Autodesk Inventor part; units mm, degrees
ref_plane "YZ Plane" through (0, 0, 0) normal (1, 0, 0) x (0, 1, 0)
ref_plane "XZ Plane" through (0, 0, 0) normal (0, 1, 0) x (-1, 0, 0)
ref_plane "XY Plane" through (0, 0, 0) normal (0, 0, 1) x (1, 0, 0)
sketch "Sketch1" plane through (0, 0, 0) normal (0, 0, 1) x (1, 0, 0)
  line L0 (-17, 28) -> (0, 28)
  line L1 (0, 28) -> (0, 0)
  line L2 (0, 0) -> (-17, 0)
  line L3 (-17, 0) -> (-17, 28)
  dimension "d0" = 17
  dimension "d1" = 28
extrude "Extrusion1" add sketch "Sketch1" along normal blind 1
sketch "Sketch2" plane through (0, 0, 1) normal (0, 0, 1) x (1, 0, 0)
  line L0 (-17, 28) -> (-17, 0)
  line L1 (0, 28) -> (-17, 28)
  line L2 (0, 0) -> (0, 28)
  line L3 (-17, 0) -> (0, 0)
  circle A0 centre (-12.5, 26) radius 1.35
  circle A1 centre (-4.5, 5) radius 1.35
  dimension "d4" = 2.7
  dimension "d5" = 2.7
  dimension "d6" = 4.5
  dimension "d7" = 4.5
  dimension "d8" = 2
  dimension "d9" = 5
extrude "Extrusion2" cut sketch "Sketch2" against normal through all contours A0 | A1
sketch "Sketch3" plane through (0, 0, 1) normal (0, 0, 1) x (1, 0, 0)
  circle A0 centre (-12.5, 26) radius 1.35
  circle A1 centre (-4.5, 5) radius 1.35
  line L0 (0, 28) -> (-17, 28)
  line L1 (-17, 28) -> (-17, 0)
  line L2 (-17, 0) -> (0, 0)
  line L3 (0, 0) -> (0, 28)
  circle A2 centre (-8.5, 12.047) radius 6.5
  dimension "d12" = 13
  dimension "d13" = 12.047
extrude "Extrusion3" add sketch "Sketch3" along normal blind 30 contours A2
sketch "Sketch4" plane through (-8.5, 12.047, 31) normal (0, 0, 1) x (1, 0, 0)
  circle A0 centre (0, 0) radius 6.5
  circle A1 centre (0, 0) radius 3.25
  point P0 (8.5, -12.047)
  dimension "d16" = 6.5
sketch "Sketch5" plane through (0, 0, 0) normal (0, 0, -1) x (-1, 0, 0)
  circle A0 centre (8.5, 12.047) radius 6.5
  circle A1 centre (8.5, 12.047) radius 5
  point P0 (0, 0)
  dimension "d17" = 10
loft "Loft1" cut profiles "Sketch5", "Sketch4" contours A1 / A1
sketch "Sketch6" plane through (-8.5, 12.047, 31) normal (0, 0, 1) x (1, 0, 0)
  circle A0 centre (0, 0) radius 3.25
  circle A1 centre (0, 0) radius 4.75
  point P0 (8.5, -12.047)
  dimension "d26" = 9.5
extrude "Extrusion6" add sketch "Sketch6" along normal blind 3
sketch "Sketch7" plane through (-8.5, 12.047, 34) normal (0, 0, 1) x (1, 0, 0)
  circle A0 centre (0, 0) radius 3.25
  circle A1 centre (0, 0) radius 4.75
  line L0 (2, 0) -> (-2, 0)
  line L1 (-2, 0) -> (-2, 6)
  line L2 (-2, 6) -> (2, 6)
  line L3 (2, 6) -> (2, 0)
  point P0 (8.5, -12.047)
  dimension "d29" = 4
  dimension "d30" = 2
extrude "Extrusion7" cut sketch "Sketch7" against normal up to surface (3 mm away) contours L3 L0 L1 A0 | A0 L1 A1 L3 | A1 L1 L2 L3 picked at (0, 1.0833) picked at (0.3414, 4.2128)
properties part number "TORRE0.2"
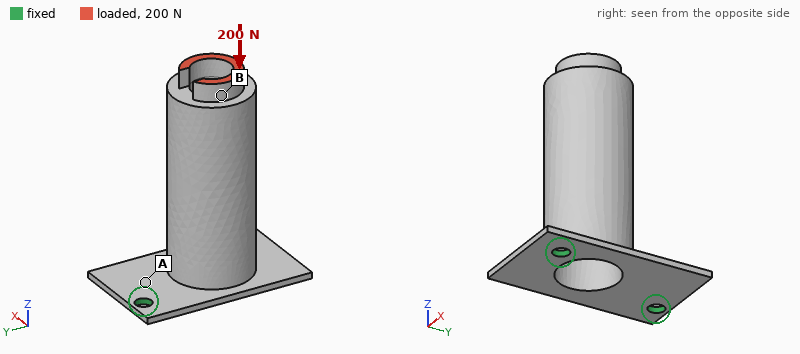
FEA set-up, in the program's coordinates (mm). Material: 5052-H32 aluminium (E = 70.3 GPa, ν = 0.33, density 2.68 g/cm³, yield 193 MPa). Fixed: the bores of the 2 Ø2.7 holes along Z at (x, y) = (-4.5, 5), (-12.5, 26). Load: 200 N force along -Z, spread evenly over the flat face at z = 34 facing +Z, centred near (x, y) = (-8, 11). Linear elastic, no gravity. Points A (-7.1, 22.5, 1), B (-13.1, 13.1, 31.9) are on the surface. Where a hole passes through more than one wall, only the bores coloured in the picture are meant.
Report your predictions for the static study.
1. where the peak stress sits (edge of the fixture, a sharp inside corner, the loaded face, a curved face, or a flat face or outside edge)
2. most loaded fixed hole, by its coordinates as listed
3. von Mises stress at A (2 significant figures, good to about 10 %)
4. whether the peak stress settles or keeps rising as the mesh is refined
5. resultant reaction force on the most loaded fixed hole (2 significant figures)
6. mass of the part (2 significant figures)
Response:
edge of the fixture
(-4.5, 5)
35 MPa
keeps rising
140 N
7.7 g
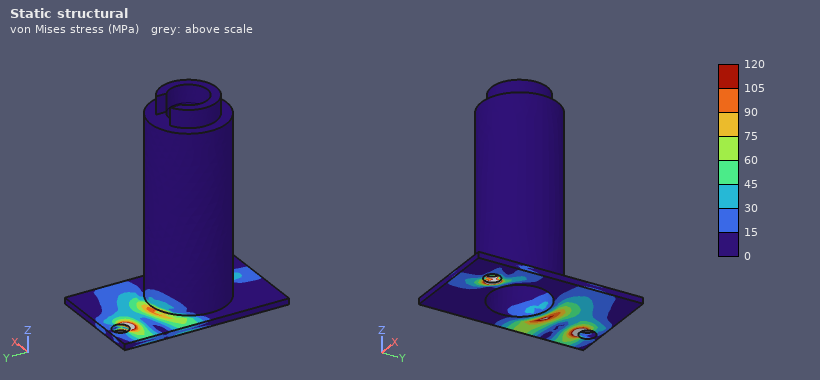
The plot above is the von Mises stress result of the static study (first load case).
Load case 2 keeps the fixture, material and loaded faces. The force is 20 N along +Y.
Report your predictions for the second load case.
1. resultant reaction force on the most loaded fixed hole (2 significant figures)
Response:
34 N
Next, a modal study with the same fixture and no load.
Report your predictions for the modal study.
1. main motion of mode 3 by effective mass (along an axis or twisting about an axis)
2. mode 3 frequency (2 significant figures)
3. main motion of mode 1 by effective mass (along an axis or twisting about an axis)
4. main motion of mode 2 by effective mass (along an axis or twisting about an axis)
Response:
along Z
11 kHz
along X
along Y
